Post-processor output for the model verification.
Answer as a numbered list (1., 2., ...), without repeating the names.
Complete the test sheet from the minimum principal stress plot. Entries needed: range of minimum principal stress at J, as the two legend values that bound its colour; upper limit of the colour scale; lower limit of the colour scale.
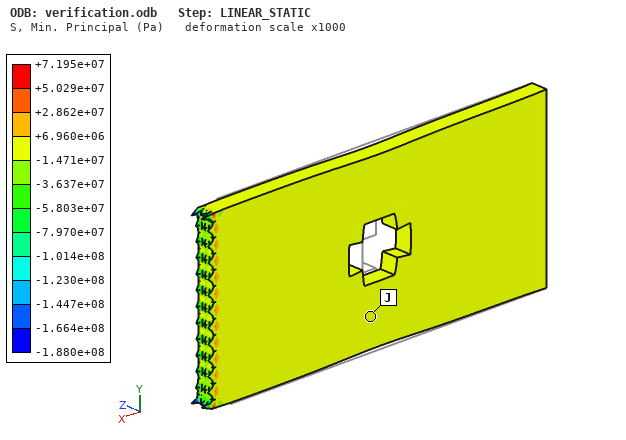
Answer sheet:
1. -1.471e+07 to +6.960e+06 Pa
2. +7.195e+07 Pa
3. -1.880e+08 Pa
